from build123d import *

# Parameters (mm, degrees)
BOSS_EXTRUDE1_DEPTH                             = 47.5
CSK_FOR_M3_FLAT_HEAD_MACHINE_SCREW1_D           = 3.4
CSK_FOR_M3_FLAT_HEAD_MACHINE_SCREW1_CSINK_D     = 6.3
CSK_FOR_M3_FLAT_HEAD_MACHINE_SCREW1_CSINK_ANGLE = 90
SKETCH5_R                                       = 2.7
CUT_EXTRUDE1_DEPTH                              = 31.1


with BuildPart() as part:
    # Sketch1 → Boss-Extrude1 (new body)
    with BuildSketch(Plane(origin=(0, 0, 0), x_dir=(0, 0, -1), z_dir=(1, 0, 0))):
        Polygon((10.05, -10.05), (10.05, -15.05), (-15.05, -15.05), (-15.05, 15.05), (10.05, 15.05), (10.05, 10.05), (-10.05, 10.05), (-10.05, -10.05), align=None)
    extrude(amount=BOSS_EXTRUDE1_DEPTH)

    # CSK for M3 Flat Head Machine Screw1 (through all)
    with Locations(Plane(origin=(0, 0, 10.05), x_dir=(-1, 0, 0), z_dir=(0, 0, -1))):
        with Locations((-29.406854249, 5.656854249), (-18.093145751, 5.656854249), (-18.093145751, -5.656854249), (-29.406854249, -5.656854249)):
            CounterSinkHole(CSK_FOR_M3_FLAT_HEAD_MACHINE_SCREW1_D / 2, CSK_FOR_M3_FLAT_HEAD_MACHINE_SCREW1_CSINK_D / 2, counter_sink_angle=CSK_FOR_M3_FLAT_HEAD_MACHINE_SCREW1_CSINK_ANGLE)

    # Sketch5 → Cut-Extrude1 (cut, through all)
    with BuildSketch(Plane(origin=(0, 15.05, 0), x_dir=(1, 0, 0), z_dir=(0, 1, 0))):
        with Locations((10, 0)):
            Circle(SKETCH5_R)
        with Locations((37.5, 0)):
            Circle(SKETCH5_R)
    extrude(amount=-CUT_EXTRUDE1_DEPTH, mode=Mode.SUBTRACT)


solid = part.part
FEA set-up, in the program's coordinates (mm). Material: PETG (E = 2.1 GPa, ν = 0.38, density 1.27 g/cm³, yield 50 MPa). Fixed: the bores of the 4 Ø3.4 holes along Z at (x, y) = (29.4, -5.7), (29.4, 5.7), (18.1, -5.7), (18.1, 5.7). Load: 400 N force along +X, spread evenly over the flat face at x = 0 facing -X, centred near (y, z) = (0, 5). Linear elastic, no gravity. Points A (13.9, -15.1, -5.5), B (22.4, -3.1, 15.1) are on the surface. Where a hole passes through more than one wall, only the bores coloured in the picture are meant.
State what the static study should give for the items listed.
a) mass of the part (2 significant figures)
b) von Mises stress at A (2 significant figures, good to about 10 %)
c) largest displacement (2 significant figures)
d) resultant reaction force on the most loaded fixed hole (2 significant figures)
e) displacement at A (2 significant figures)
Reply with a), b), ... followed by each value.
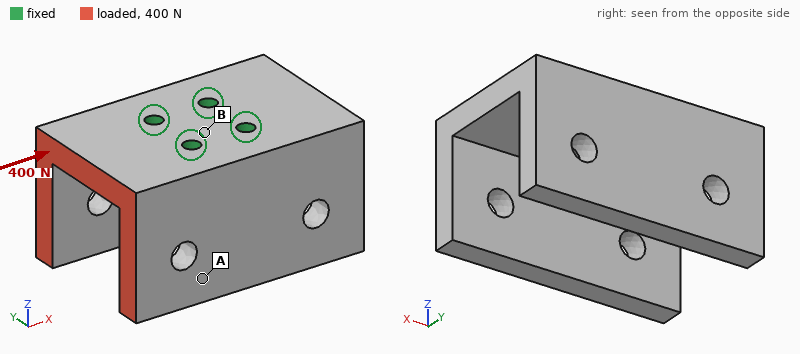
a) 20 g
b) 1.8 MPa
c) 0.18 mm
d) 160 N
e) 0.11 mm
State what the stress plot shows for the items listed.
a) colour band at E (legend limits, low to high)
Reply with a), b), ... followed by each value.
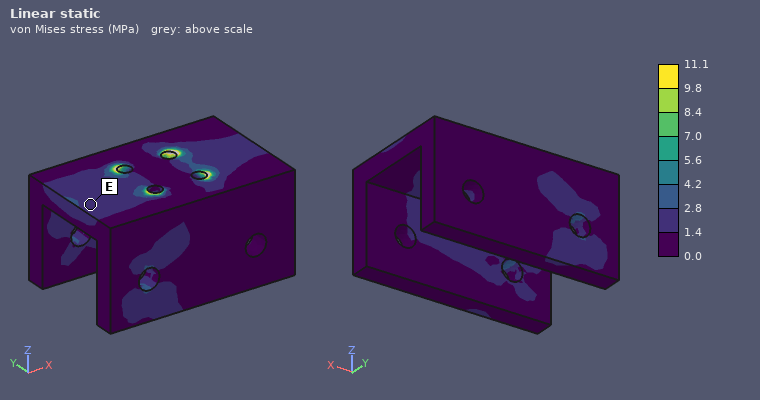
a) 1.4 to 2.8 MPa
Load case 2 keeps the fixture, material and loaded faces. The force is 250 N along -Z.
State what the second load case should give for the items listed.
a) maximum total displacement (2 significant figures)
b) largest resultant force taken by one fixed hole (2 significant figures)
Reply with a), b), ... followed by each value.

a) 0.36 mm
b) 250 N
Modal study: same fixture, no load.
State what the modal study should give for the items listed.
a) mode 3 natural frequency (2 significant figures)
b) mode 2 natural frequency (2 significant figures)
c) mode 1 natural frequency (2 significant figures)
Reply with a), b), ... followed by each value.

a) 1700 Hz
b) 1300 Hz
c) 1300 Hz
